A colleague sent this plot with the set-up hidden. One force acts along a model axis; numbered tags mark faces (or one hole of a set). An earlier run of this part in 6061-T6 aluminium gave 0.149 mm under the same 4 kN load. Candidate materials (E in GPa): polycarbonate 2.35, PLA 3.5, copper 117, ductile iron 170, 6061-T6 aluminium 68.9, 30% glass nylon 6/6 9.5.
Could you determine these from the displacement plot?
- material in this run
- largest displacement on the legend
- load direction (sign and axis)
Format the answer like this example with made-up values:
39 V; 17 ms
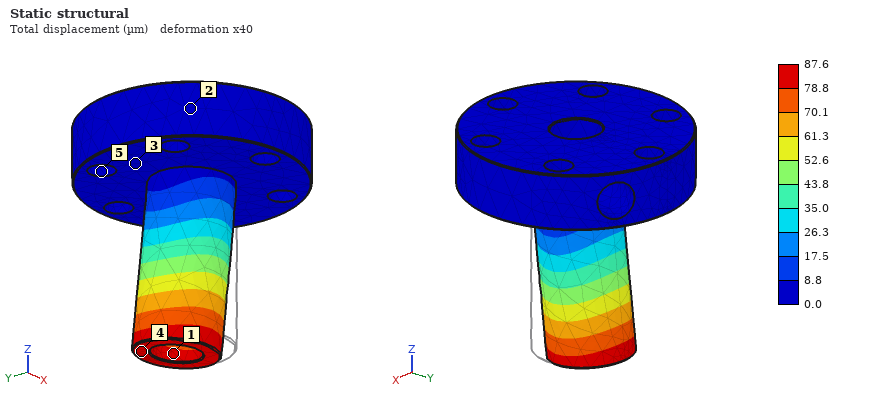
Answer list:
copper; 87.6 µm; +Y
